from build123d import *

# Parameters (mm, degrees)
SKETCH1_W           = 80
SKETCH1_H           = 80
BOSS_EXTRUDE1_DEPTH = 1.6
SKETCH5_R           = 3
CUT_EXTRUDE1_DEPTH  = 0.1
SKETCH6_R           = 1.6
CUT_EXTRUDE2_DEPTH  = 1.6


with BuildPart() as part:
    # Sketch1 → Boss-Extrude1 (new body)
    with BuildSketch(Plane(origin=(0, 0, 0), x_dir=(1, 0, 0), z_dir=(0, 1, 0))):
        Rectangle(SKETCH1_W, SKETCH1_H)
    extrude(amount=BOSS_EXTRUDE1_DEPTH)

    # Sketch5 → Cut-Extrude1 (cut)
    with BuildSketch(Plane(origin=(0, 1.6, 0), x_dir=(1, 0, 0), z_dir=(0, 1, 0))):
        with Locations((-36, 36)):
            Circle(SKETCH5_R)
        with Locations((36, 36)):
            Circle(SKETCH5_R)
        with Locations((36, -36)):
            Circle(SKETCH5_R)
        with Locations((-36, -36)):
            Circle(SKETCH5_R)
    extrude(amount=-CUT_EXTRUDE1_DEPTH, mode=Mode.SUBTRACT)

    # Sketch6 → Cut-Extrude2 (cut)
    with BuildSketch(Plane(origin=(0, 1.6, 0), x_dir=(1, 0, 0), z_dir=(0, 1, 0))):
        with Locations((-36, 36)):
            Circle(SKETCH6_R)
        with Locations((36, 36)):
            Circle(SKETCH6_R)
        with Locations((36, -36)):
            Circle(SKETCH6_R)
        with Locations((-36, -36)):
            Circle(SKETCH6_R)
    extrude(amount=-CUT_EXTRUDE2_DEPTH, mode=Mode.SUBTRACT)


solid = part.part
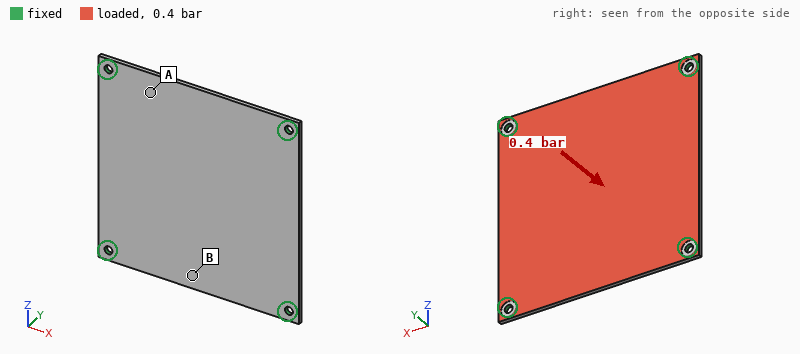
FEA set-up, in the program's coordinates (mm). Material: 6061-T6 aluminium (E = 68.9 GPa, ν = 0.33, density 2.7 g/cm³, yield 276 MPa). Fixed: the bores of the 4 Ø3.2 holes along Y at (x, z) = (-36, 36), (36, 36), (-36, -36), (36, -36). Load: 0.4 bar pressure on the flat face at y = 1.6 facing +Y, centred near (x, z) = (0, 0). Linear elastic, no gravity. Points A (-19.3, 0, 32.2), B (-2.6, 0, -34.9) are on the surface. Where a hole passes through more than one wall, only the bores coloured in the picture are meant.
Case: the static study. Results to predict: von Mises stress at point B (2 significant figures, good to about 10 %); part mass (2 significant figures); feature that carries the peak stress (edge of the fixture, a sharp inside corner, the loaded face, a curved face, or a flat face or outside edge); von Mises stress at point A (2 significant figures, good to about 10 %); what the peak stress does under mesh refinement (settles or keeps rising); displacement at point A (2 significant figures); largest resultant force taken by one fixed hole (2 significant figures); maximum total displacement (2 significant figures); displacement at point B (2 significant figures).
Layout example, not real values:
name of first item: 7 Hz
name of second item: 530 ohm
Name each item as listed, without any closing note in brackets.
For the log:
von Mises stress at point B: 29 MPa
part mass: 27 g
feature that carries the peak stress: edge of the fixture
von Mises stress at point A: 11 MPa
what the peak stress does under mesh refinement: keeps rising
displacement at point A: 0.12 mm
largest resultant force taken by one fixed hole: 64 N
maximum total displacement: 0.34 mm
displacement at point B: 0.19 mm
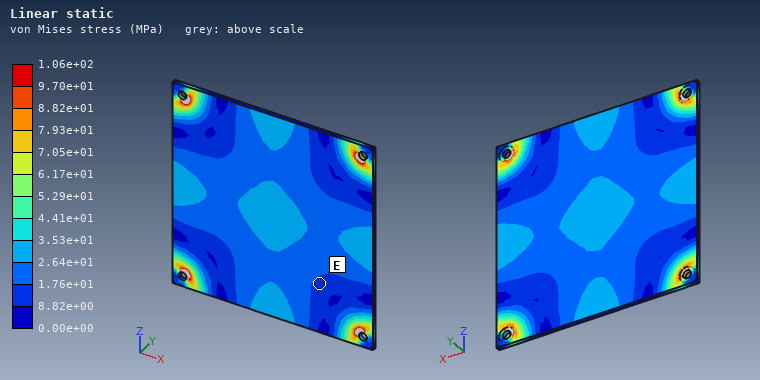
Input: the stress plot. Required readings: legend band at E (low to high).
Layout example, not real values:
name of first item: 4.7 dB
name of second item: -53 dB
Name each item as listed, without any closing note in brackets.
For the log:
legend band at E: 8.82e+00 to 1.76e+01 MPa
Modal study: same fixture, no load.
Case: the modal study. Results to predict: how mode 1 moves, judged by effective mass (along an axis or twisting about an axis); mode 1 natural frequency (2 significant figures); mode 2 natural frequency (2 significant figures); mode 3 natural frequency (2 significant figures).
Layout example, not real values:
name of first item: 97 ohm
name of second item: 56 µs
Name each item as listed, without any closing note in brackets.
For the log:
how mode 1 moves, judged by effective mass: along Y
mode 1 natural frequency: 1000 Hz
mode 2 natural frequency: 1800 Hz
mode 3 natural frequency: 1800 Hz
